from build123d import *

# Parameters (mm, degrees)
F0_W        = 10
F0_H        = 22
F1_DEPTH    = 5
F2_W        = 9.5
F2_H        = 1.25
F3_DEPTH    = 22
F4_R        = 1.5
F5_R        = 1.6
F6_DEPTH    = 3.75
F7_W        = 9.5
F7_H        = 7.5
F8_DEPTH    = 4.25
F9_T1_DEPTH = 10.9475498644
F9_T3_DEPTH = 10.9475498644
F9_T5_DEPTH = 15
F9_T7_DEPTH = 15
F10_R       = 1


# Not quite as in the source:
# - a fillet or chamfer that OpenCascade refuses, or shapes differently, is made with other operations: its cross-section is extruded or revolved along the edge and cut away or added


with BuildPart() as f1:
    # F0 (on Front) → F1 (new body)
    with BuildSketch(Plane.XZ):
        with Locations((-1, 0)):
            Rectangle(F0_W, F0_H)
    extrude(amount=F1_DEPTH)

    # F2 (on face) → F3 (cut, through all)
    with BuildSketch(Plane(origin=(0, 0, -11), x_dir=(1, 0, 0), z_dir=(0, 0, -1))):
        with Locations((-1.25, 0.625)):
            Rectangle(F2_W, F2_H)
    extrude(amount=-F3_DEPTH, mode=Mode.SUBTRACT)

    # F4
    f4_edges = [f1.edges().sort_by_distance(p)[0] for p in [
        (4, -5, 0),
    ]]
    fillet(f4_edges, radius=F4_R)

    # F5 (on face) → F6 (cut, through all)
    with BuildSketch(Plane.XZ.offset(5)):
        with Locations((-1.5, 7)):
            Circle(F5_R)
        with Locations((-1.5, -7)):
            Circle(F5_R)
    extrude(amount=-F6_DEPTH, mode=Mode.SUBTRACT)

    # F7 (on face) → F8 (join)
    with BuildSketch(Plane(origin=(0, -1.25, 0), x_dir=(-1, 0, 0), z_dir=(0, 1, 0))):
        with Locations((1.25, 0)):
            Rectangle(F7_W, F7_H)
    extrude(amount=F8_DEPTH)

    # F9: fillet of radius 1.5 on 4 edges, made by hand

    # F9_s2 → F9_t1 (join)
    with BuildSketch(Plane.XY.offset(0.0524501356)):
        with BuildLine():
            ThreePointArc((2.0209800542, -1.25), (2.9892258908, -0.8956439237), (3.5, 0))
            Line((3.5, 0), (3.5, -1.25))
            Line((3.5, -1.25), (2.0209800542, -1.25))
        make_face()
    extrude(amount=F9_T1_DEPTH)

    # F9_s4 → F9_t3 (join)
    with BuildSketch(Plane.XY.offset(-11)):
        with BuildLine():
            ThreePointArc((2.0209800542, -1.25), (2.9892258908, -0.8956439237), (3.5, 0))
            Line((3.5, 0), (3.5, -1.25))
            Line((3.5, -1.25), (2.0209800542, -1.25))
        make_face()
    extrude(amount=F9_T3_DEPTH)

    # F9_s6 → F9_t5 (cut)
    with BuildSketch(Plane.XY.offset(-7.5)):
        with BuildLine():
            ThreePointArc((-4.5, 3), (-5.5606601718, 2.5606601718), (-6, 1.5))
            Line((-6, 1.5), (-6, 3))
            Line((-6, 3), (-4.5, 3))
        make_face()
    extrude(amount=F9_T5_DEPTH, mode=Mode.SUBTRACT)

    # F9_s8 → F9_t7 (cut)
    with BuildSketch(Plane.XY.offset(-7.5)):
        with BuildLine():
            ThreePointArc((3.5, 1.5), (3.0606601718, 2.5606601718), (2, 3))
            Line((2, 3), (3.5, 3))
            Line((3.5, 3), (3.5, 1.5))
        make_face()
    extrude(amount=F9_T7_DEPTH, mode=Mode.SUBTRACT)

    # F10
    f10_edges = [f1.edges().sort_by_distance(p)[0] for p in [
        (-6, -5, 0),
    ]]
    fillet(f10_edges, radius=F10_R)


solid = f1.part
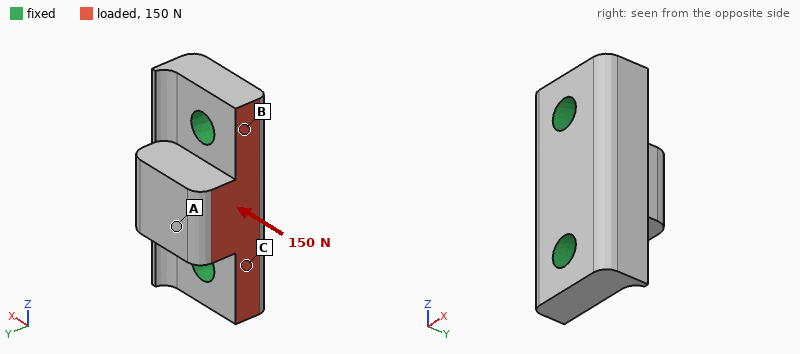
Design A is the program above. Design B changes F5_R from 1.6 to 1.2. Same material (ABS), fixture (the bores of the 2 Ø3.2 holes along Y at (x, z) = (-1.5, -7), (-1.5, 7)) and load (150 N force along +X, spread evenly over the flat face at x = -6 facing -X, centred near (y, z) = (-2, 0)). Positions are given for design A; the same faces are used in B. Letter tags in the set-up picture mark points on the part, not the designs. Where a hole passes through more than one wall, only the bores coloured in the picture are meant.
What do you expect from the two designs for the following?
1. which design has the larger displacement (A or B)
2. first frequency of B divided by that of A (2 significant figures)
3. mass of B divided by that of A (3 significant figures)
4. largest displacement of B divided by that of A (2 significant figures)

B
0.89
1.02
1.2
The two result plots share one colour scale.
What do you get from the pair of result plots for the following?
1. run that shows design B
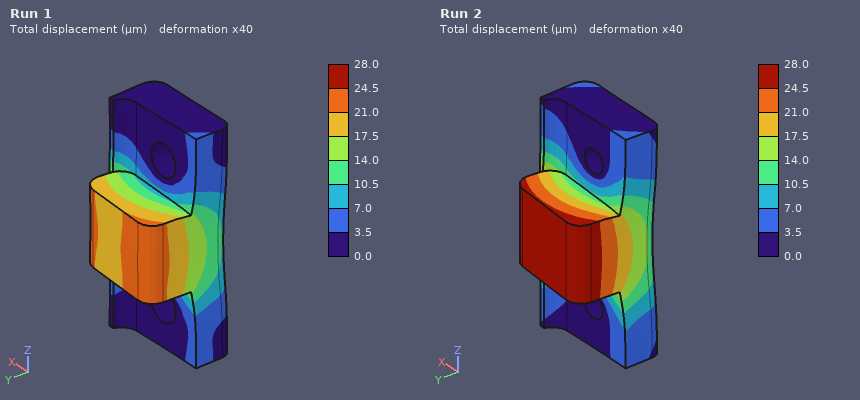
Run 2
